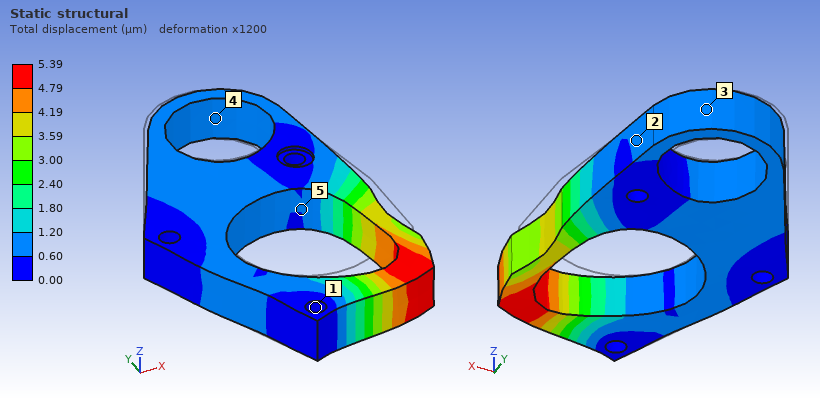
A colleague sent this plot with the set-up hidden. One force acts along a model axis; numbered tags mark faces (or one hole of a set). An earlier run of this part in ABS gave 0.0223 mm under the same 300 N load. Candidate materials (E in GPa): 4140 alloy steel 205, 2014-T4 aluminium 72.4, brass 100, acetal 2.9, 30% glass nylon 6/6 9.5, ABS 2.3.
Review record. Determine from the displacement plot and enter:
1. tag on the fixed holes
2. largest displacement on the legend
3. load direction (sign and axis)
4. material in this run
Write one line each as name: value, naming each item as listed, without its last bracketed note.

tag on the fixed holes: 1
largest displacement on the legend: 5.39 µm
load direction: -Y
material in this run: 30% glass nylon 6/6
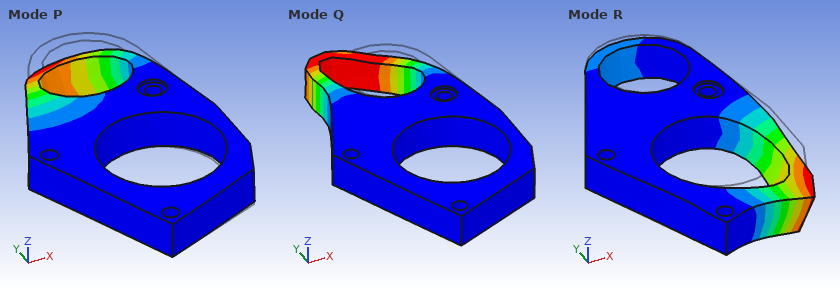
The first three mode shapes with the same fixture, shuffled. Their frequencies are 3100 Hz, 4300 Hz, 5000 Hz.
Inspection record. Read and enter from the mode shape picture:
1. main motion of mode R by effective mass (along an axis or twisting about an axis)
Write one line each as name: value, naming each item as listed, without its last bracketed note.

main motion of mode R by effective mass: along Z
